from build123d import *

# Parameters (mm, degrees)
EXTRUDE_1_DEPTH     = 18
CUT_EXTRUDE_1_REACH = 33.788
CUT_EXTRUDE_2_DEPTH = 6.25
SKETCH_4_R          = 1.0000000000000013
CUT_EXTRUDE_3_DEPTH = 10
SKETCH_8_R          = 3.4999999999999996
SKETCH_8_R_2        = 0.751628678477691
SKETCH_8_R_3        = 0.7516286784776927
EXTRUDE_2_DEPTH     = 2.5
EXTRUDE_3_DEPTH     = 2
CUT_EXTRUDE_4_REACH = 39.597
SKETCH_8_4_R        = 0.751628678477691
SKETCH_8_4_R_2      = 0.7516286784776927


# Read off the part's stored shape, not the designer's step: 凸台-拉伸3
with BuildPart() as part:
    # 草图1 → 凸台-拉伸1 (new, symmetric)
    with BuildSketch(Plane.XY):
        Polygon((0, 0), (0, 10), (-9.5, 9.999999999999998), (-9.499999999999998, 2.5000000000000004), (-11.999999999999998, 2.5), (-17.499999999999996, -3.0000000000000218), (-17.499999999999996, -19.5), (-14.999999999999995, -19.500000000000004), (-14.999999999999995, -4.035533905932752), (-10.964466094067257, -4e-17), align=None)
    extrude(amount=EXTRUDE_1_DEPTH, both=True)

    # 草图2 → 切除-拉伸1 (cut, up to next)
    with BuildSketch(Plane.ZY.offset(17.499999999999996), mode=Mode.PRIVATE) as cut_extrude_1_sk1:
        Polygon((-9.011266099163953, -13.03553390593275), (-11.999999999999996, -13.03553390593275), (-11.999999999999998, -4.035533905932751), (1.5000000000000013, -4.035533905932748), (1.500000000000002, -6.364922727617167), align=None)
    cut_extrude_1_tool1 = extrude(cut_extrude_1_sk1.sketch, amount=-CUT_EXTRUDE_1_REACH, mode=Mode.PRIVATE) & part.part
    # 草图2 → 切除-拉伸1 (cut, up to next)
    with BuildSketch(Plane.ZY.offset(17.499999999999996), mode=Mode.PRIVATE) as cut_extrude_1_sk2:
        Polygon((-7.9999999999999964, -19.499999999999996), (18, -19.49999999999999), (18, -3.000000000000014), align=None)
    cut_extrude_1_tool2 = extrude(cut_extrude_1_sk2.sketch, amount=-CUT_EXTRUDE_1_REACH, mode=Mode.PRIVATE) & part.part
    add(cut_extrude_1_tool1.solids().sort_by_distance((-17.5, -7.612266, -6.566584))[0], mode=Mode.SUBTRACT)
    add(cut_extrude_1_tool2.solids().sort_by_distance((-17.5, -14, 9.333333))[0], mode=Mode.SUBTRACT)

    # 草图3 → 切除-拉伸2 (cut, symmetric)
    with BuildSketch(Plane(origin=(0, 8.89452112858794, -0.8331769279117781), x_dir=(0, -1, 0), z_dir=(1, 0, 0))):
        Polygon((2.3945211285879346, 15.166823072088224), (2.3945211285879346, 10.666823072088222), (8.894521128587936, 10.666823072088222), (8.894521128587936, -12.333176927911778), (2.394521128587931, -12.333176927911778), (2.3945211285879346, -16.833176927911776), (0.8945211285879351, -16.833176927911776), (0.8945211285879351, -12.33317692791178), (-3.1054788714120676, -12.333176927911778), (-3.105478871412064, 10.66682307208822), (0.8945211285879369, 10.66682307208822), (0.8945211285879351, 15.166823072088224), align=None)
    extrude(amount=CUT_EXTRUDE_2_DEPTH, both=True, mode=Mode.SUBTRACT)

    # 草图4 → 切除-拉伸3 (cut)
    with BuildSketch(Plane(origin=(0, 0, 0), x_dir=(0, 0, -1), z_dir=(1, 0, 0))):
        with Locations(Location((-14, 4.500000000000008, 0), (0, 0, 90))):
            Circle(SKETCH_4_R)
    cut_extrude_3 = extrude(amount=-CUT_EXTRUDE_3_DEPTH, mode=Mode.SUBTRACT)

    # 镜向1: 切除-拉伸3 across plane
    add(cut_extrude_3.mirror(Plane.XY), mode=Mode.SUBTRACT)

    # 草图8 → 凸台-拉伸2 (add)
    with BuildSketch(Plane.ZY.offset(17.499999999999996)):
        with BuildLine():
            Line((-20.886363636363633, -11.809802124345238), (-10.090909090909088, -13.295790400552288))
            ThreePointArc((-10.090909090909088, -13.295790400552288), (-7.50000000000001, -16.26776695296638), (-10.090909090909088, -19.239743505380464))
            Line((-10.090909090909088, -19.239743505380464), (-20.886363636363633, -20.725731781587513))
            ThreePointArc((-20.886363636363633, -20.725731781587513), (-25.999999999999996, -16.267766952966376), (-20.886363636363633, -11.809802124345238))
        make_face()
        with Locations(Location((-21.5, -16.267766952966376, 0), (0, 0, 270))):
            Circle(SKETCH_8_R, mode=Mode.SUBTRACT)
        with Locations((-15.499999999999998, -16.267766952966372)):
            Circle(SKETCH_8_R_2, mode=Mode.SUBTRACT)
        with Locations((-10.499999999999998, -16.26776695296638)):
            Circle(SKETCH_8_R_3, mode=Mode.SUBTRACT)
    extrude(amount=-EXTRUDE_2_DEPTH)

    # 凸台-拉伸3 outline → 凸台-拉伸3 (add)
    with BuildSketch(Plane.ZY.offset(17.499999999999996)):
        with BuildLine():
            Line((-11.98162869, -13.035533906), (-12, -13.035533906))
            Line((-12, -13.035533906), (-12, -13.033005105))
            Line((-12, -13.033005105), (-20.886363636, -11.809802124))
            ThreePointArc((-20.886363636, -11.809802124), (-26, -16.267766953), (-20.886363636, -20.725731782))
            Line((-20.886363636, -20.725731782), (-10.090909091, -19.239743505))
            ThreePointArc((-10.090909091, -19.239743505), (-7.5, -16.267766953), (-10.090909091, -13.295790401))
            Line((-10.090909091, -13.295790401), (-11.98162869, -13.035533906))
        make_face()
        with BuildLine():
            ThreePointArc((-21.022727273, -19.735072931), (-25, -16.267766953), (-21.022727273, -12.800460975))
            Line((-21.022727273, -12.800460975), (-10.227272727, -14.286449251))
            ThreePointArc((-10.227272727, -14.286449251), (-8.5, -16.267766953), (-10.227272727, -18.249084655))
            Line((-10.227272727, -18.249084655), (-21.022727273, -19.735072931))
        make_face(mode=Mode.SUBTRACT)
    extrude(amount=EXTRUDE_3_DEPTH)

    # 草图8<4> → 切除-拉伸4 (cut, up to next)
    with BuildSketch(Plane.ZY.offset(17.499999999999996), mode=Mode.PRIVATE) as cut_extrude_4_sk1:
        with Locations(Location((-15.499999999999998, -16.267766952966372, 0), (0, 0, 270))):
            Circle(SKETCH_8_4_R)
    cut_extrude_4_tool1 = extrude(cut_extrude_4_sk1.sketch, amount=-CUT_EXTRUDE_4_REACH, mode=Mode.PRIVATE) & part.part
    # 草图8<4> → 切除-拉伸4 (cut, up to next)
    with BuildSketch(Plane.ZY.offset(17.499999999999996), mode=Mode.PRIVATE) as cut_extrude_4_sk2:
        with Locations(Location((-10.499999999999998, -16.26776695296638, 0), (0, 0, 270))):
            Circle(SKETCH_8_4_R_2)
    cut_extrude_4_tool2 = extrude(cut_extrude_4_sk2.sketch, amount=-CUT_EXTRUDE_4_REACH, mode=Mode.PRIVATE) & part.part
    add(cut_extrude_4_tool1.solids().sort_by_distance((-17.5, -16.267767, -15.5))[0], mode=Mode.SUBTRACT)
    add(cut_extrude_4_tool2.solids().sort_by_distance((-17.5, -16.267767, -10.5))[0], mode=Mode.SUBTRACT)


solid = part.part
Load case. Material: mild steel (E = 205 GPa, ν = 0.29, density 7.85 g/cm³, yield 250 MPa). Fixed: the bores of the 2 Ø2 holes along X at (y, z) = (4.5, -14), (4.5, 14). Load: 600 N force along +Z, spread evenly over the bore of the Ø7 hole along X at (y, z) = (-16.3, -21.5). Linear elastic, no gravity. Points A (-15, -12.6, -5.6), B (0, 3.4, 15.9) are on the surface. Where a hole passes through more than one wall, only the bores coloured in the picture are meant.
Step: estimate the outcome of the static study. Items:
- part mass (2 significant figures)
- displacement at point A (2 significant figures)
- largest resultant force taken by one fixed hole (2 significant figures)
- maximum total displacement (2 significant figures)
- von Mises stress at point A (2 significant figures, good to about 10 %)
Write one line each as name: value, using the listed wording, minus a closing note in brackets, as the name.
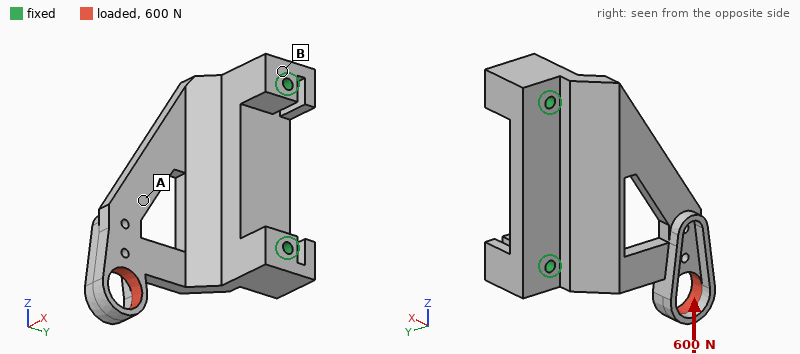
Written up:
part mass: 27 g
displacement at point A: 20 µm
largest resultant force taken by one fixed hole: 560 N
maximum total displacement: 70 µm
von Mises stress at point A: 53 MPa
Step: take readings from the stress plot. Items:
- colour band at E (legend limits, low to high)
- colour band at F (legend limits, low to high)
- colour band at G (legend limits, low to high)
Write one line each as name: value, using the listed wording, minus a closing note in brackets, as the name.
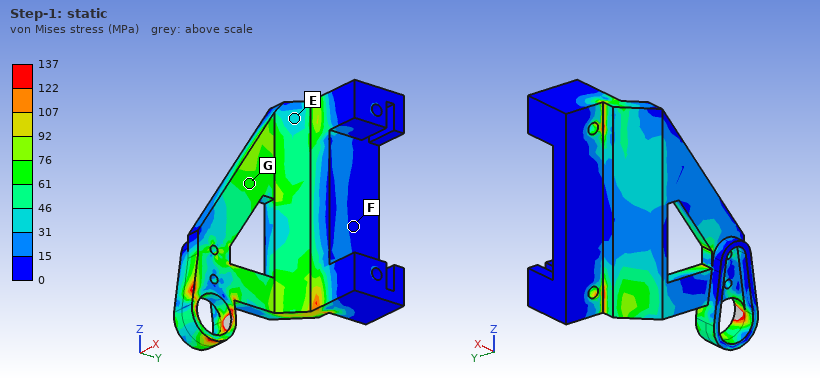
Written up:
colour band at E: 31 to 46 MPa
colour band at F: 0 to 15 MPa
colour band at G: 61 to 76 MPa
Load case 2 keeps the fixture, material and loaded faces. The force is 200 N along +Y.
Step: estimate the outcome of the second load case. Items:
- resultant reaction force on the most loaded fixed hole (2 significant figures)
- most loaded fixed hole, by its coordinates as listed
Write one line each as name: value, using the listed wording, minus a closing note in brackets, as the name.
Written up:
resultant reaction force on the most loaded fixed hole: 250 N
most loaded fixed hole, by its coordinates as listed: (4.5, -14)
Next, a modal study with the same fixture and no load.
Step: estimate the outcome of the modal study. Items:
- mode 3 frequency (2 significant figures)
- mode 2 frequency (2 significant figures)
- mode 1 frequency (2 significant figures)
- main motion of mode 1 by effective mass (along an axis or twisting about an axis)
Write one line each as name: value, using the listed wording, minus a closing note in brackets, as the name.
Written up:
mode 3 frequency: 10 kHz
mode 2 frequency: 7700 Hz
mode 1 frequency: 3000 Hz
main motion of mode 1 by effective mass: along X
